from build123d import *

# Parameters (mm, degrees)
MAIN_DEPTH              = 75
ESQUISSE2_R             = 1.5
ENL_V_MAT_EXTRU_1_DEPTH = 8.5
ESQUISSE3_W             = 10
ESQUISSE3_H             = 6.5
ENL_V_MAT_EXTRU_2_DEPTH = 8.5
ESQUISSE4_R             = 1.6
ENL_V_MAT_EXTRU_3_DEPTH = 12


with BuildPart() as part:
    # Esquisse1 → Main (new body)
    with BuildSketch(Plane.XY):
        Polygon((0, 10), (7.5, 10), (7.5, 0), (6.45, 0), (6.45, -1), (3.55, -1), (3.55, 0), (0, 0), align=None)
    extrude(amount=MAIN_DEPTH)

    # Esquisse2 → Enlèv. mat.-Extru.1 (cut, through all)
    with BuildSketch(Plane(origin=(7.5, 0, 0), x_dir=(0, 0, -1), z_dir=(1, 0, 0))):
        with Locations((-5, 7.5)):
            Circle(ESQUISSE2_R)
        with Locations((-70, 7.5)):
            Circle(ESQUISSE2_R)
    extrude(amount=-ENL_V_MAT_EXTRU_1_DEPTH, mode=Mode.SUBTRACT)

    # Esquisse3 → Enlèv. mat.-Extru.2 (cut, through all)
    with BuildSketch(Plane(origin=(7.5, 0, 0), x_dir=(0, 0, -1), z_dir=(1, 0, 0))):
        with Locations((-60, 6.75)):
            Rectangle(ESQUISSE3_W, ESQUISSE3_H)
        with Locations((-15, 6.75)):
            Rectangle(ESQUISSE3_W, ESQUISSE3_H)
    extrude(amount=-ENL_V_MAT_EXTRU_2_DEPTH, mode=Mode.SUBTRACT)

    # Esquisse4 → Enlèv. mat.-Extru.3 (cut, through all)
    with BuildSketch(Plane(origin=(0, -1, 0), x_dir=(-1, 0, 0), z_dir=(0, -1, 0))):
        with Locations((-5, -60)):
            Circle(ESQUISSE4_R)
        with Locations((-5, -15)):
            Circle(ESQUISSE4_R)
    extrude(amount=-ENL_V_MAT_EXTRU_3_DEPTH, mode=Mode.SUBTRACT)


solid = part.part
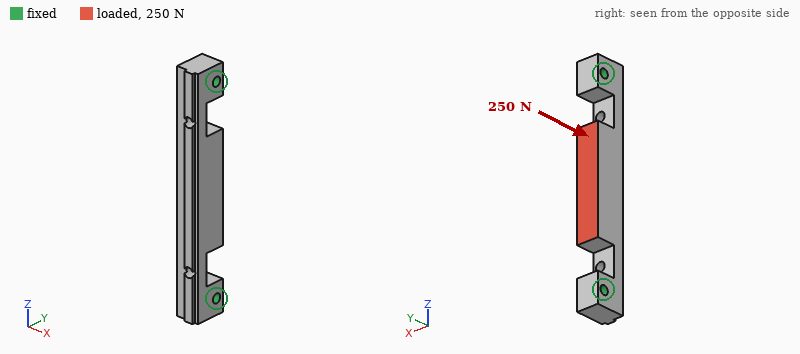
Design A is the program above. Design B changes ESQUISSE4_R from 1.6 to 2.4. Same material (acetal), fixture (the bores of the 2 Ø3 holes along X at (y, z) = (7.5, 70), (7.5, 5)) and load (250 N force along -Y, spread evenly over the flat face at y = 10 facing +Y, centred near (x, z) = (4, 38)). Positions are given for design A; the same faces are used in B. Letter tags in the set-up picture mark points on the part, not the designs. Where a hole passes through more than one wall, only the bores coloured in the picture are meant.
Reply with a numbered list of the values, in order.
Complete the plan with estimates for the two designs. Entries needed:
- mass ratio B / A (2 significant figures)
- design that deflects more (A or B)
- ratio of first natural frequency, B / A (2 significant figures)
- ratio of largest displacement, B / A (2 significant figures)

1. 0.98
2. B
3. 0.87
4. 1.3
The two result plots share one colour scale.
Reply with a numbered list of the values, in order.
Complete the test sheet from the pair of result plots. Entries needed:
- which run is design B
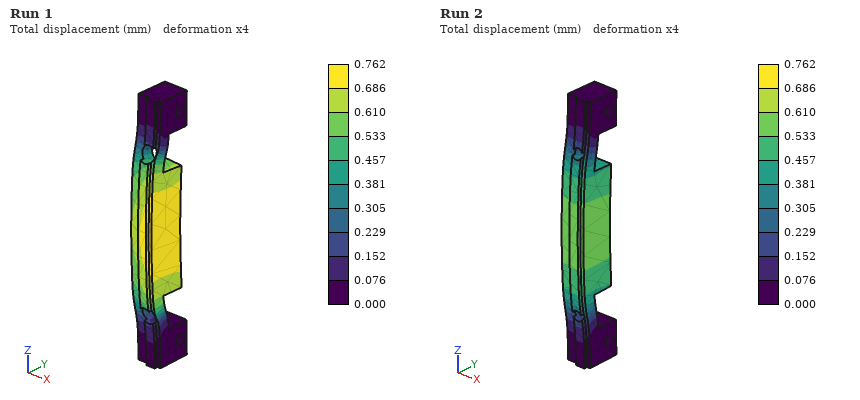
1. Run 1
